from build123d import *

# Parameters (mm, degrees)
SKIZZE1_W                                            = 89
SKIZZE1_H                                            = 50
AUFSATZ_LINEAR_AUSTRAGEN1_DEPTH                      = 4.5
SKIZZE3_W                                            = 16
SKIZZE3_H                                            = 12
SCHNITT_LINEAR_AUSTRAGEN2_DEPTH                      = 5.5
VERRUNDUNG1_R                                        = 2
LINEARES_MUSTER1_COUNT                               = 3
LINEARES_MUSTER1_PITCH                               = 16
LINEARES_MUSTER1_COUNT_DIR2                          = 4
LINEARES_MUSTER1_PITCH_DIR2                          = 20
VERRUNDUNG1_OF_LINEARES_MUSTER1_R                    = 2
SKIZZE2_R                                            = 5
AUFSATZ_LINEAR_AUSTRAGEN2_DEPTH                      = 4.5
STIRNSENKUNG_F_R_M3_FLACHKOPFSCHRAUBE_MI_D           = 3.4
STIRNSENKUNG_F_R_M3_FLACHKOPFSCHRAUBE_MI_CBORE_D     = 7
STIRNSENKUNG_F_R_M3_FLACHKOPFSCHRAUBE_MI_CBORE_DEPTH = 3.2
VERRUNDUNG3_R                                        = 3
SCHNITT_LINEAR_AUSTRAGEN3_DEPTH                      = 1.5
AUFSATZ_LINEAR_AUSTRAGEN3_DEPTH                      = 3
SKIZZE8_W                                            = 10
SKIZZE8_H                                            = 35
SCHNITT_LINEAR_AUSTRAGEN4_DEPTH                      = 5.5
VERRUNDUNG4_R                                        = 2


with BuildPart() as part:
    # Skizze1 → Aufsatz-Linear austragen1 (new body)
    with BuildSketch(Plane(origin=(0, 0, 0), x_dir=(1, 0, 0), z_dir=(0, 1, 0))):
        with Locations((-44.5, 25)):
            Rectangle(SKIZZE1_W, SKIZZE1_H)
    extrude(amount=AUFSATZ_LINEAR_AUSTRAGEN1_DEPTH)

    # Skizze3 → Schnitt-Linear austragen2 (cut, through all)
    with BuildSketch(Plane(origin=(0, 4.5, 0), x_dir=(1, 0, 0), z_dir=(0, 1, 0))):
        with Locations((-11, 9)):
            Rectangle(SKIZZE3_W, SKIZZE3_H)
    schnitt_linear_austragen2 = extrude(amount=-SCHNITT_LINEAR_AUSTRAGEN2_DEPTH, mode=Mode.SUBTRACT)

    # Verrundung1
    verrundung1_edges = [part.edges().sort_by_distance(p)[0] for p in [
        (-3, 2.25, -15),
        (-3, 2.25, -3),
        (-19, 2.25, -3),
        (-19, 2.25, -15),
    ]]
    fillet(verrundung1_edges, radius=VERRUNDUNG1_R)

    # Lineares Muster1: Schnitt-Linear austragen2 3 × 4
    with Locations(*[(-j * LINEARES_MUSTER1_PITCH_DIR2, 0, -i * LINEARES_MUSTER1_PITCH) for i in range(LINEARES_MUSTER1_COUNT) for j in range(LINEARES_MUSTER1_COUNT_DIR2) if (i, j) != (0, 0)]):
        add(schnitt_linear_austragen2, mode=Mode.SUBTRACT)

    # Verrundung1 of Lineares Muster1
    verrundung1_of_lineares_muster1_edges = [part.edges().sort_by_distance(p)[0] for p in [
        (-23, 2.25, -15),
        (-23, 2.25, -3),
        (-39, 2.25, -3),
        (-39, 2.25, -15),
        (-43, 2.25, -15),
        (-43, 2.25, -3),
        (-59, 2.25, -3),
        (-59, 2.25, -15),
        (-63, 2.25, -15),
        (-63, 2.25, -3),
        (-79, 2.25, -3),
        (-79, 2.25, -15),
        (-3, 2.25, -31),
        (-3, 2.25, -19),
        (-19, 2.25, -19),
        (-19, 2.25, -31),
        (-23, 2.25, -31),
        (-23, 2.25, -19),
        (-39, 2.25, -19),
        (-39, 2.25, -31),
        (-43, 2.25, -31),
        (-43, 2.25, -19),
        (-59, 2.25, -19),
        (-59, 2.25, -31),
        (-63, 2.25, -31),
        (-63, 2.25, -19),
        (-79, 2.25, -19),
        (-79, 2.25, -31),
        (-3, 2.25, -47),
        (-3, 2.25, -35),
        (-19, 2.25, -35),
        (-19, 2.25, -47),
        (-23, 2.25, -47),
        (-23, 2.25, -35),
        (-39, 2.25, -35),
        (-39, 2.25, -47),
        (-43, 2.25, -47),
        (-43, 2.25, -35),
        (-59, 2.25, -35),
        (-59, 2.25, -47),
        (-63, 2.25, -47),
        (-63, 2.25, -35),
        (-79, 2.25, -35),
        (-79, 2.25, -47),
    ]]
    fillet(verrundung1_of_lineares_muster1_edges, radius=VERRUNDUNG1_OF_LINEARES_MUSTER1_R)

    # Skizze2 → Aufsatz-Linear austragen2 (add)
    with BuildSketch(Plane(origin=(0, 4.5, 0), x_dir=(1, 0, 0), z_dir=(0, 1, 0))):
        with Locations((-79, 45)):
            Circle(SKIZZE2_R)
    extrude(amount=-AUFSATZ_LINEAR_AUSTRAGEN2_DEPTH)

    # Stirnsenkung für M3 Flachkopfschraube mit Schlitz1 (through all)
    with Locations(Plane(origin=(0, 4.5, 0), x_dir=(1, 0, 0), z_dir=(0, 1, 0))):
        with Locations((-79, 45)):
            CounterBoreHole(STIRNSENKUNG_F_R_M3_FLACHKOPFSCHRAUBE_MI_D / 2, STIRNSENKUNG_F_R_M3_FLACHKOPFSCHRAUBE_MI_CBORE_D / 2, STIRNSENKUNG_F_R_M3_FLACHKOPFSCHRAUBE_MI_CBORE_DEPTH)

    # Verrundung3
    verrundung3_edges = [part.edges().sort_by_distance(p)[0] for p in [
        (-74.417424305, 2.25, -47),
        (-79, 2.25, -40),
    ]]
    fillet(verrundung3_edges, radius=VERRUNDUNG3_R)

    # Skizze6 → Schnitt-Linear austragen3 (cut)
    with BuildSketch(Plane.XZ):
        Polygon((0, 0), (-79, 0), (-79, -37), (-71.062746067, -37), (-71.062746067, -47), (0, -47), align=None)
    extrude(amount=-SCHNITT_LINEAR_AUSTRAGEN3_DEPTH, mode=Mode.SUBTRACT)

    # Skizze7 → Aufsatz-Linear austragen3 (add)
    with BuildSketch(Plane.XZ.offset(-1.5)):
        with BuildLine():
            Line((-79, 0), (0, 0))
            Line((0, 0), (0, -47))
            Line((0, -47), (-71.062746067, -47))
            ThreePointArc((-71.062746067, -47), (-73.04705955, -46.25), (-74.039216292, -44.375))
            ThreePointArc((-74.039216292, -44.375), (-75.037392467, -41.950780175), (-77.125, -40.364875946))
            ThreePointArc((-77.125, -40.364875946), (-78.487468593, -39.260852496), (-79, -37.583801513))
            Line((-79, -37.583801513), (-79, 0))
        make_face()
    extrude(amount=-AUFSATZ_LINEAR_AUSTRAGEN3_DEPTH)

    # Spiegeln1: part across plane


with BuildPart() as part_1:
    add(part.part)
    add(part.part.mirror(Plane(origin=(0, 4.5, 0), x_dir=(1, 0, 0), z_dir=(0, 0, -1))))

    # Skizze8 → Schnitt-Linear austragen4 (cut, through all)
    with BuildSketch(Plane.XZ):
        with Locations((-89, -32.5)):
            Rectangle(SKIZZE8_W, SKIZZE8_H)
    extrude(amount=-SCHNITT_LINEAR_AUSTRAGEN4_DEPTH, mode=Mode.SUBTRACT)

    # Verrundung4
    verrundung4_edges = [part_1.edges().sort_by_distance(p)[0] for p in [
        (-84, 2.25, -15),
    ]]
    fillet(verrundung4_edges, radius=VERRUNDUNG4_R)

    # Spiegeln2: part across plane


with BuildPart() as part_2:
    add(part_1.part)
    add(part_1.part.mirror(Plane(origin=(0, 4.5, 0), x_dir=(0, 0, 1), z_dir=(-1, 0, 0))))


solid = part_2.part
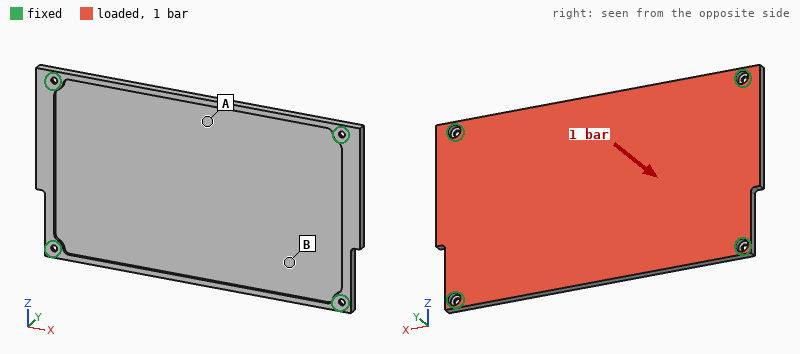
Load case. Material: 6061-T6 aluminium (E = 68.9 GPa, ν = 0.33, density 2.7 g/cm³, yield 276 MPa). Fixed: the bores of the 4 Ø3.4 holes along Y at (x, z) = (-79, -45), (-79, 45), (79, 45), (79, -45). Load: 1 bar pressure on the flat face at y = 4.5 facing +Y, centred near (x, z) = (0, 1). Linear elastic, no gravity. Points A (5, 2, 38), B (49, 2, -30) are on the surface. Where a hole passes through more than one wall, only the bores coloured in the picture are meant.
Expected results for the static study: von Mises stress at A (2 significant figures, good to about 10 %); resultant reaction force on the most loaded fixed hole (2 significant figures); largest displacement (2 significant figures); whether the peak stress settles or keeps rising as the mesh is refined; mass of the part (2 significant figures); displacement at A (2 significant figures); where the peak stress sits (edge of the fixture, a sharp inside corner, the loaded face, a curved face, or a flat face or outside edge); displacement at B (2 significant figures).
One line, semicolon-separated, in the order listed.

54 MPa; 2.2 kN; 1.4 mm; keeps rising; 150 g; 1.4 mm; edge of the fixture; 0.68 mm
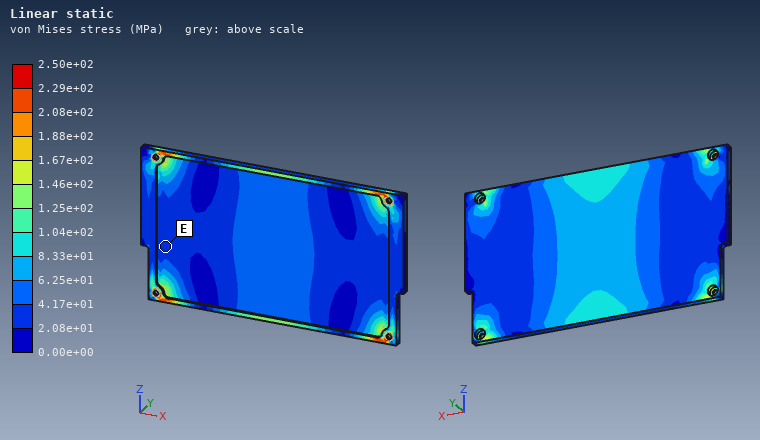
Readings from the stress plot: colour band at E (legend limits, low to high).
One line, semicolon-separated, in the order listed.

2.08e+01 to 4.17e+01 MPa
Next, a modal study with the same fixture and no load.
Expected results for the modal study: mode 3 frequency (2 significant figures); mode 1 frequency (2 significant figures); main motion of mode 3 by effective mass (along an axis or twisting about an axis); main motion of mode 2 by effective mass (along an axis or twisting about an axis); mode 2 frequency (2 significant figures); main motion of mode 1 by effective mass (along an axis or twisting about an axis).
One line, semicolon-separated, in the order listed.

1300 Hz; 530 Hz; twisting about Z; twisting about X; 900 Hz; along Y
